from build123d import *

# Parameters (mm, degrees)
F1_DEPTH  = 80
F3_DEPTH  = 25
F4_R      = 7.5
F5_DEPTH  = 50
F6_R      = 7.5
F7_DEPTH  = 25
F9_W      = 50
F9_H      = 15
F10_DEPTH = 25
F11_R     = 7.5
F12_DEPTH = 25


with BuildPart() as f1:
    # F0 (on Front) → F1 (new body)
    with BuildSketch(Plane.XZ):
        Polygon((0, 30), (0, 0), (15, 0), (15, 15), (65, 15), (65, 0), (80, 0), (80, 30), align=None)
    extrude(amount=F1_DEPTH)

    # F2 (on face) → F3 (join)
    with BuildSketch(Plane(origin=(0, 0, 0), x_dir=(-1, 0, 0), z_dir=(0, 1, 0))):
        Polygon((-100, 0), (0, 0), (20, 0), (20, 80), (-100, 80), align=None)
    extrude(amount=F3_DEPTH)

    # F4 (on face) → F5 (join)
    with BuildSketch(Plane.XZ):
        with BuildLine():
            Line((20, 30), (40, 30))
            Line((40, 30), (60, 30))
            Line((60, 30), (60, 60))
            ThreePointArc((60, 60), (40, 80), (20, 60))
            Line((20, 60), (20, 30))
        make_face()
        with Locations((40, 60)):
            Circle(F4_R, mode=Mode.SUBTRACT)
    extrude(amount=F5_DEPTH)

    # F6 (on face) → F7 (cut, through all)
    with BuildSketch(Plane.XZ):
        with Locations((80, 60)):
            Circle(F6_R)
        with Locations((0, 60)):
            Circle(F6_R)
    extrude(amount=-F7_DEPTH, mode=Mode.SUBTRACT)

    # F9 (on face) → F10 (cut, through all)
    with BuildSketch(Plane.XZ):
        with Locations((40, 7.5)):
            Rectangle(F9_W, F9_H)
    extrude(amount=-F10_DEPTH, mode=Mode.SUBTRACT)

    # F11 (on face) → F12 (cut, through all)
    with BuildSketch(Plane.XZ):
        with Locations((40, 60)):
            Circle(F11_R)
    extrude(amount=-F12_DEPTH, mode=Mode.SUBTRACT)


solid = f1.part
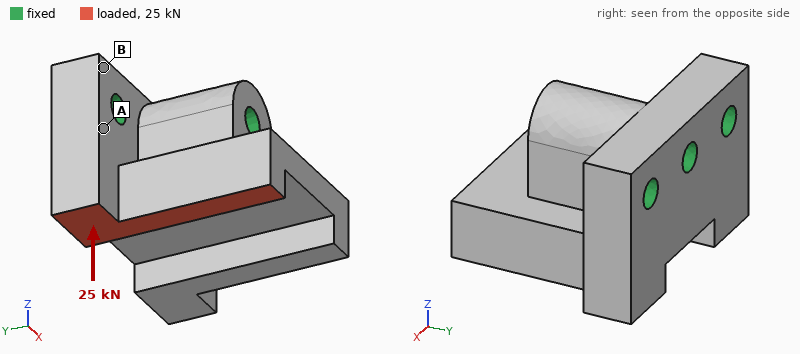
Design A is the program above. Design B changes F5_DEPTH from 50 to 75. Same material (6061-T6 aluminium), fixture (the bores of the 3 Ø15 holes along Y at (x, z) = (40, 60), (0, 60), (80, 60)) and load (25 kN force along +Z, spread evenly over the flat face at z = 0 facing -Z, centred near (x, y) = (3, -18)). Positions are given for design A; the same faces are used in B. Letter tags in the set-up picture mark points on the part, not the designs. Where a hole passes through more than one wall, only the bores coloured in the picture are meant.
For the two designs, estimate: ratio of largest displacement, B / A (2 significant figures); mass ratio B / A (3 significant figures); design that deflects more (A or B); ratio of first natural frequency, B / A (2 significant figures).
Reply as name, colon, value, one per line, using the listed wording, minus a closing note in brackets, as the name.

ratio of largest displacement, B / A: 0.57
mass ratio B / A: 1.10
design that deflects more: A
ratio of first natural frequency, B / A: 1.2
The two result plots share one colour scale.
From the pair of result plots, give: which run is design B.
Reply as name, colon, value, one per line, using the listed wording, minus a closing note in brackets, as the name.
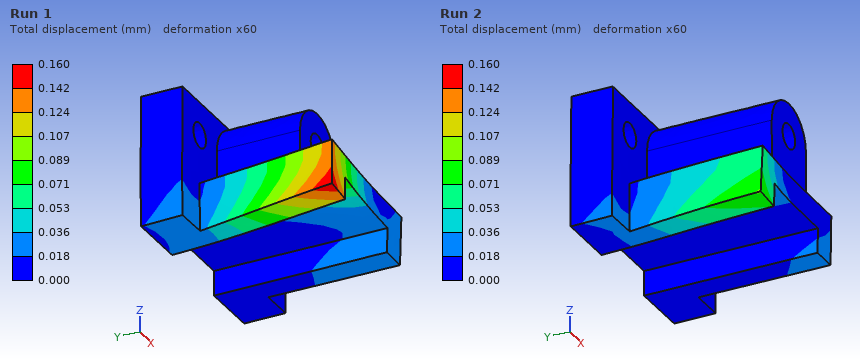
which run is design B: Run 2
